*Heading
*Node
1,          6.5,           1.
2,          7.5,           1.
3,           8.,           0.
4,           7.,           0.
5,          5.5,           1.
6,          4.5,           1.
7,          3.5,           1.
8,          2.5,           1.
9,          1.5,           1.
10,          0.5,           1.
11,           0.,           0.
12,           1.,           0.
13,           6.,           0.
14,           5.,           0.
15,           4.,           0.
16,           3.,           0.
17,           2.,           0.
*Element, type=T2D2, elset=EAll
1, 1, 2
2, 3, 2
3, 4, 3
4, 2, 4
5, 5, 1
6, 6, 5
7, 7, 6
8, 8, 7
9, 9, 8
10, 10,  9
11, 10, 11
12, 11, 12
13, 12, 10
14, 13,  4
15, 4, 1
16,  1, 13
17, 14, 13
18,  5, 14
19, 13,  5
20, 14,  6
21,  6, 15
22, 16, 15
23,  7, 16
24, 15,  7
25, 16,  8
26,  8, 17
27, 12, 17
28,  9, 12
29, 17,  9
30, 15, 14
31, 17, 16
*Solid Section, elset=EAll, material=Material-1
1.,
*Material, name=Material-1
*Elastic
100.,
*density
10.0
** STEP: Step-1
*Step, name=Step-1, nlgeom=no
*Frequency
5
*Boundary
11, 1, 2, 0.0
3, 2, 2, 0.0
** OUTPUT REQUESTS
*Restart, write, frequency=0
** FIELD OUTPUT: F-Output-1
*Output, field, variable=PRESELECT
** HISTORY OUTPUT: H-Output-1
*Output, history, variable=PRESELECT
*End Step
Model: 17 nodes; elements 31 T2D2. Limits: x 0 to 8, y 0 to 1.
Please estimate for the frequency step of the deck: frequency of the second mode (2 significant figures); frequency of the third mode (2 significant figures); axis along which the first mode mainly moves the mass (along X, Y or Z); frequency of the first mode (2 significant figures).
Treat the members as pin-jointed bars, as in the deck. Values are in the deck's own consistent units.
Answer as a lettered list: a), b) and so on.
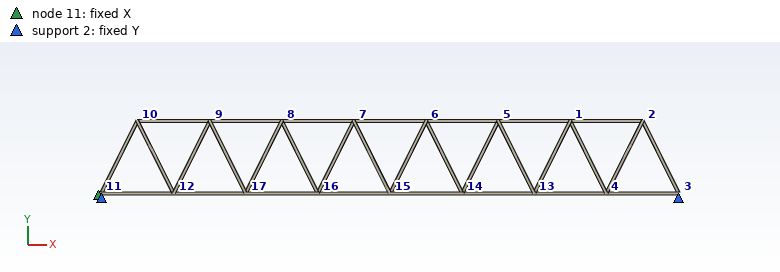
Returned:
a) 0.058 cycles per unit time
b) 0.082 cycles per unit time
c) along Y
d) 0.023 cycles per unit time
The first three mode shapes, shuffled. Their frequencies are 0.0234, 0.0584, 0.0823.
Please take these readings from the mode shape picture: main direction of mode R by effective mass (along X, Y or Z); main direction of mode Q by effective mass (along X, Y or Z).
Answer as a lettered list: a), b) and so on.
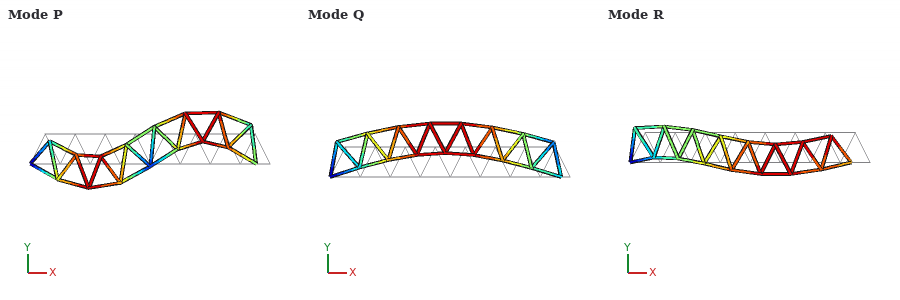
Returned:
a) along X
b) along Y
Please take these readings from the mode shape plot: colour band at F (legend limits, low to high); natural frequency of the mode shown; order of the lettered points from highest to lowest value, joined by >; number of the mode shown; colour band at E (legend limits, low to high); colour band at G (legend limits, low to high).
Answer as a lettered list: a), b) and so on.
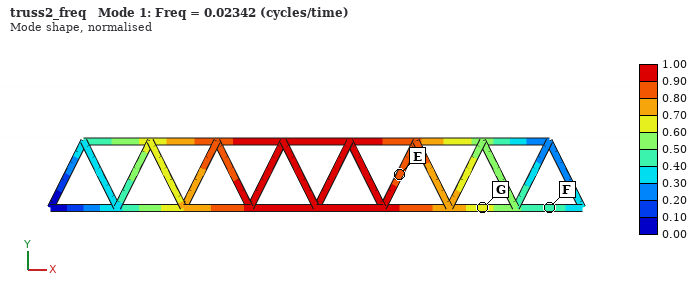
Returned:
a) 0.40 to 0.50
b) 0.02342
c) E > G > F
d) 1
e) 0.80 to 0.90
f) 0.60 to 0.70
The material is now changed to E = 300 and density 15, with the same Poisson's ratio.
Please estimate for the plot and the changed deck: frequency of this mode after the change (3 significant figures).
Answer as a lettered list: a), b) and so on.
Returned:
a) 0.0331
